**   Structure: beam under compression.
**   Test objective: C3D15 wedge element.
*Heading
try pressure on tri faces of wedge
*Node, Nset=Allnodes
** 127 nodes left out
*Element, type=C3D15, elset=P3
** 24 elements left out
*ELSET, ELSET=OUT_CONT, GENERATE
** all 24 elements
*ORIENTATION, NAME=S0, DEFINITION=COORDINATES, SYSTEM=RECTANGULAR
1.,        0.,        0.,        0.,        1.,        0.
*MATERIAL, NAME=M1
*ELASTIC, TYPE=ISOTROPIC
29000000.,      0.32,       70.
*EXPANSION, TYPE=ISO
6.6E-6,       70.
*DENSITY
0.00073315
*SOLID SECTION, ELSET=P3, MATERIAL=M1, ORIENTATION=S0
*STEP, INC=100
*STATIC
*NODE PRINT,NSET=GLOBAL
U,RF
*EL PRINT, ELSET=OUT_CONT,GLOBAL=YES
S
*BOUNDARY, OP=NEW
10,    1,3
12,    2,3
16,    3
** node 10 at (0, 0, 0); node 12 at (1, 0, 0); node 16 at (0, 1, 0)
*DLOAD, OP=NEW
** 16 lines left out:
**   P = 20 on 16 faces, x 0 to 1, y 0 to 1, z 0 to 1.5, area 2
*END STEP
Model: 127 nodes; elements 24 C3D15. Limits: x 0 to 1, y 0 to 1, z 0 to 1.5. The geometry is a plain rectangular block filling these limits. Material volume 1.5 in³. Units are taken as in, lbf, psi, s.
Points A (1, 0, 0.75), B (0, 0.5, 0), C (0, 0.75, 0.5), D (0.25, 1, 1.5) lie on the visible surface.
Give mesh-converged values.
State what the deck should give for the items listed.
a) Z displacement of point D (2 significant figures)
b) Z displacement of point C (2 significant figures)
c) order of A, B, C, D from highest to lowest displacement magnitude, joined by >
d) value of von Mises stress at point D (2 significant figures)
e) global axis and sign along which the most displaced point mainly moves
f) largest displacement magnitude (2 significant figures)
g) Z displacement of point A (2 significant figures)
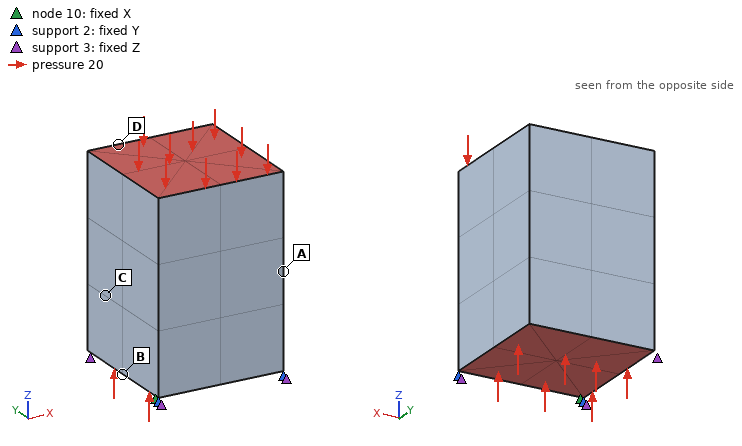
-1.0e-06 in
-3.4e-07 in
D > A > C > B
20 psi
-Z
1.1e-06 in
-5.2e-07 in
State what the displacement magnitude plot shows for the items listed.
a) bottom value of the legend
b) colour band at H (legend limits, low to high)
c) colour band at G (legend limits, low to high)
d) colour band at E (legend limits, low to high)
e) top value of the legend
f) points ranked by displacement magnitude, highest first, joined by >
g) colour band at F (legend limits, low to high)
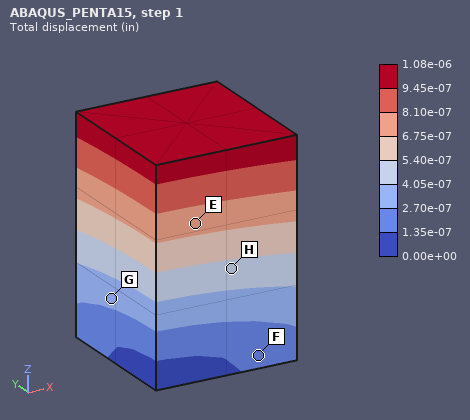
0.00e+00 in
4.05e-07 to 5.40e-07 in
2.70e-07 to 4.05e-07 in
6.75e-07 to 8.10e-07 in
1.08e-06 in
E > H > G > F
1.35e-07 to 2.70e-07 in
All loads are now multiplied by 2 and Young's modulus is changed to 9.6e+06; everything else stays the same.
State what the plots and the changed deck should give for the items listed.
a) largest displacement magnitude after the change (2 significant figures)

6.5e-06 in
